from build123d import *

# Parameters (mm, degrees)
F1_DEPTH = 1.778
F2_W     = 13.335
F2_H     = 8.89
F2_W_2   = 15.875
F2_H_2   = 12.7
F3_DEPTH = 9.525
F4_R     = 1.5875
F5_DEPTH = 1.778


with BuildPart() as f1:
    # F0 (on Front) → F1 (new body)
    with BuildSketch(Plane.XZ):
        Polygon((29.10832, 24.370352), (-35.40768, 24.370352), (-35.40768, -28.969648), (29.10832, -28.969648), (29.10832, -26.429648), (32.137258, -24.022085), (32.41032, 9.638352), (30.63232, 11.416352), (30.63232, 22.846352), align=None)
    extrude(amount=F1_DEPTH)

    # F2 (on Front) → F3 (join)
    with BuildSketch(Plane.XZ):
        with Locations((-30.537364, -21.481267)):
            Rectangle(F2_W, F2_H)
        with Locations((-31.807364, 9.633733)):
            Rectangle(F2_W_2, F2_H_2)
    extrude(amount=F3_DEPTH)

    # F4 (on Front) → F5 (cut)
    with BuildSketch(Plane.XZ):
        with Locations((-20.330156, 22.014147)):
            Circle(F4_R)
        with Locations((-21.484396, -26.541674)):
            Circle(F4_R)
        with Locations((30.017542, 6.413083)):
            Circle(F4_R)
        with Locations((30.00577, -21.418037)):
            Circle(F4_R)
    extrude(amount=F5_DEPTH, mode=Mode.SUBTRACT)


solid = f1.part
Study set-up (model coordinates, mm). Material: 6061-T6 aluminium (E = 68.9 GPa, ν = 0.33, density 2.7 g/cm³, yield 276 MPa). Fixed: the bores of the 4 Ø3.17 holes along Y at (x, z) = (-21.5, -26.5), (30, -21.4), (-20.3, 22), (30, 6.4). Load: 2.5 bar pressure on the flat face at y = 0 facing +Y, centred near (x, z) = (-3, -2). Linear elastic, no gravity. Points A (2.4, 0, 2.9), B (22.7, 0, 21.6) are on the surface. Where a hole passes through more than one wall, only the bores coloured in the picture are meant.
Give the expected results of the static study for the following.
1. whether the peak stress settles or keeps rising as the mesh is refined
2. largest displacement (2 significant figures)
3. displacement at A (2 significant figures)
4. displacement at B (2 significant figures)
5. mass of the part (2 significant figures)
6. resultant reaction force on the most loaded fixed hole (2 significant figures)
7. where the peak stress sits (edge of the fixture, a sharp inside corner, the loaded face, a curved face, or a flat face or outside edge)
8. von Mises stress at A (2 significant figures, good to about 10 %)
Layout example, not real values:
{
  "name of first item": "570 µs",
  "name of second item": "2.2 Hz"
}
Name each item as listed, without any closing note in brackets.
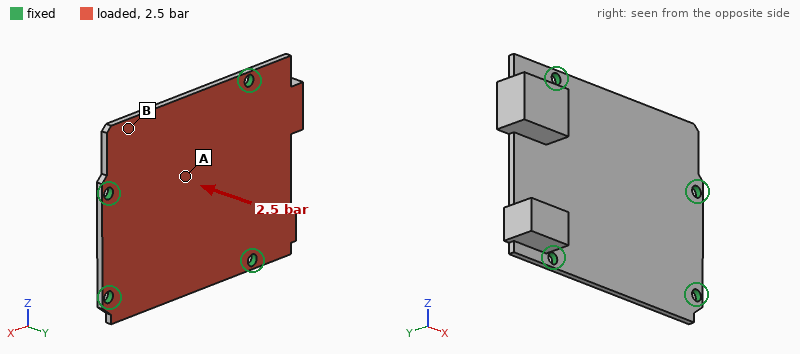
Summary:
{
  "whether the peak stress settles or keeps rising as the mesh is refined": "keeps rising",
  "largest displacement": "0.21 mm",
  "displacement at A": "0.21 mm",
  "displacement at B": "0.13 mm",
  "mass of the part": "24 g",
  "resultant reaction force on the most loaded fixed hole": "270 N",
  "where the peak stress sits": "edge of the fixture",
  "von Mises stress at A": "50 MPa"
}
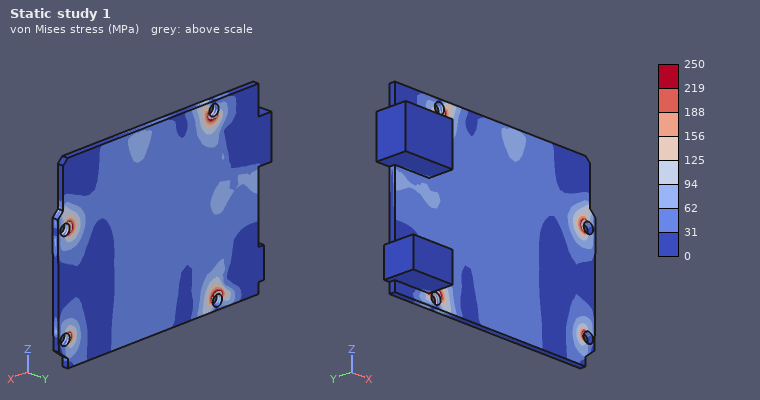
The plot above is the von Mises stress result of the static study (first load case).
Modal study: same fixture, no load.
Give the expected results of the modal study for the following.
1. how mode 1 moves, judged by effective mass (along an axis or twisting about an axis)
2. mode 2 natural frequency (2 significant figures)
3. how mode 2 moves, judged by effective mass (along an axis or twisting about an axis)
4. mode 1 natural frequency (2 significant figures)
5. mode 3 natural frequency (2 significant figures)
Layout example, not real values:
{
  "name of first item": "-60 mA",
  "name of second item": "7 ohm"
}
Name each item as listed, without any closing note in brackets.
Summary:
{
  "how mode 1 moves, judged by effective mass": "along Y",
  "mode 2 natural frequency": "2800 Hz",
  "how mode 2 moves, judged by effective mass": "along Y",
  "mode 1 natural frequency": "1900 Hz",
  "mode 3 natural frequency": "3500 Hz"
}
